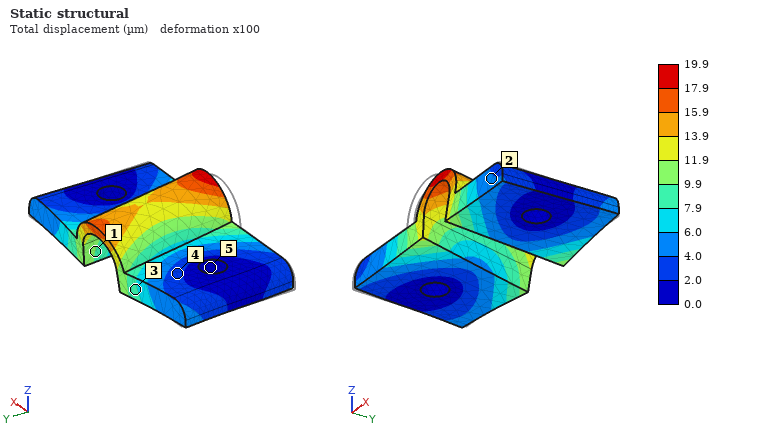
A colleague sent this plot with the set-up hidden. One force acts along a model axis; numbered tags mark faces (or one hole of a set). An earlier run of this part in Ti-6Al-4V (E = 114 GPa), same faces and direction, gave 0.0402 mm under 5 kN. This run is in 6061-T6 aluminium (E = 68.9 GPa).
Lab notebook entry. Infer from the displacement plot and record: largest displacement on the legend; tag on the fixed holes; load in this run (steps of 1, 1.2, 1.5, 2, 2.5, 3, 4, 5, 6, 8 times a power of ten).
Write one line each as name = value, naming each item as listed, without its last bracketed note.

largest displacement on the legend = 19.9 µm
tag on the fixed holes = 5
load in this run = 1.5 kN
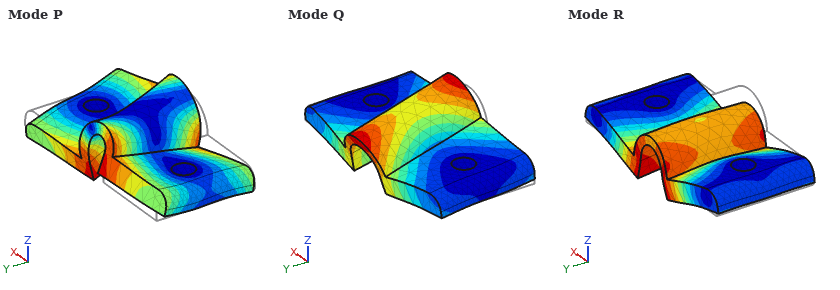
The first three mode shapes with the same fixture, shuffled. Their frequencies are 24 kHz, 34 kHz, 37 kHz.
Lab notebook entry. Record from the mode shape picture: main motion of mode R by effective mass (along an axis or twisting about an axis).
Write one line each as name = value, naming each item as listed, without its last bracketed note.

main motion of mode R by effective mass = along Z
